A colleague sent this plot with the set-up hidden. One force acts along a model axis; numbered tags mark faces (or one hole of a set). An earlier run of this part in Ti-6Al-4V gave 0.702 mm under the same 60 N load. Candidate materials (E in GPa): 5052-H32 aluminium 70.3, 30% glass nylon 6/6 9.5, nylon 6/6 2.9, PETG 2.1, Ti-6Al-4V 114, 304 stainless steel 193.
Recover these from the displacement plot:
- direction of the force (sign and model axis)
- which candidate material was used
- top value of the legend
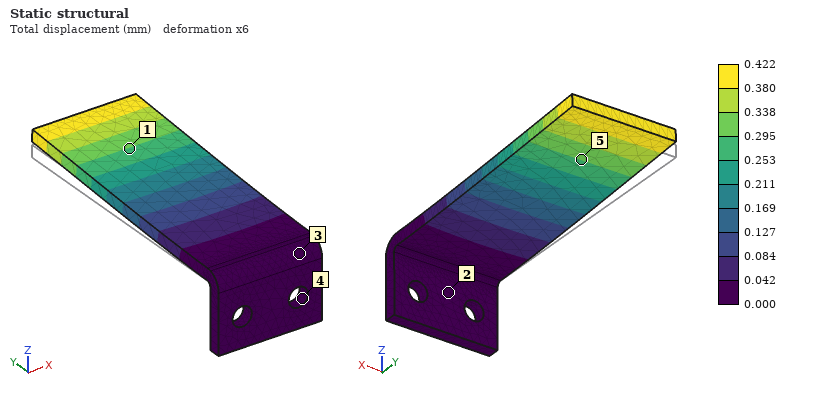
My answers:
+Z
304 stainless steel
0.422 mm
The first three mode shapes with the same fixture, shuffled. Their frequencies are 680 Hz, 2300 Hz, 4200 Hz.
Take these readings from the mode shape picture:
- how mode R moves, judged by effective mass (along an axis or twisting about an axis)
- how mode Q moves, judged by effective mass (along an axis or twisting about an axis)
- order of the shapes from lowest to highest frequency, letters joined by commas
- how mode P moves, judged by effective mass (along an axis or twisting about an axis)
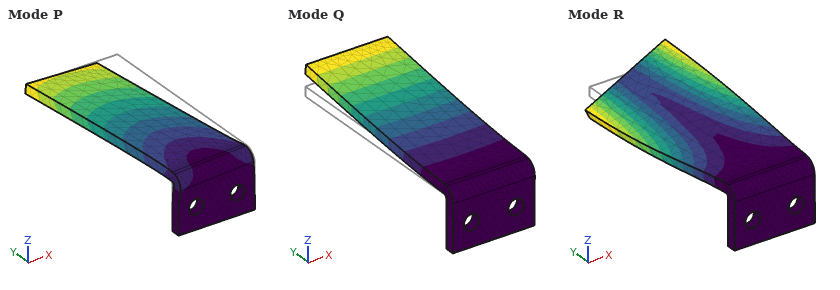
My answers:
twisting about Y
along Z
Q, P, R
along X
